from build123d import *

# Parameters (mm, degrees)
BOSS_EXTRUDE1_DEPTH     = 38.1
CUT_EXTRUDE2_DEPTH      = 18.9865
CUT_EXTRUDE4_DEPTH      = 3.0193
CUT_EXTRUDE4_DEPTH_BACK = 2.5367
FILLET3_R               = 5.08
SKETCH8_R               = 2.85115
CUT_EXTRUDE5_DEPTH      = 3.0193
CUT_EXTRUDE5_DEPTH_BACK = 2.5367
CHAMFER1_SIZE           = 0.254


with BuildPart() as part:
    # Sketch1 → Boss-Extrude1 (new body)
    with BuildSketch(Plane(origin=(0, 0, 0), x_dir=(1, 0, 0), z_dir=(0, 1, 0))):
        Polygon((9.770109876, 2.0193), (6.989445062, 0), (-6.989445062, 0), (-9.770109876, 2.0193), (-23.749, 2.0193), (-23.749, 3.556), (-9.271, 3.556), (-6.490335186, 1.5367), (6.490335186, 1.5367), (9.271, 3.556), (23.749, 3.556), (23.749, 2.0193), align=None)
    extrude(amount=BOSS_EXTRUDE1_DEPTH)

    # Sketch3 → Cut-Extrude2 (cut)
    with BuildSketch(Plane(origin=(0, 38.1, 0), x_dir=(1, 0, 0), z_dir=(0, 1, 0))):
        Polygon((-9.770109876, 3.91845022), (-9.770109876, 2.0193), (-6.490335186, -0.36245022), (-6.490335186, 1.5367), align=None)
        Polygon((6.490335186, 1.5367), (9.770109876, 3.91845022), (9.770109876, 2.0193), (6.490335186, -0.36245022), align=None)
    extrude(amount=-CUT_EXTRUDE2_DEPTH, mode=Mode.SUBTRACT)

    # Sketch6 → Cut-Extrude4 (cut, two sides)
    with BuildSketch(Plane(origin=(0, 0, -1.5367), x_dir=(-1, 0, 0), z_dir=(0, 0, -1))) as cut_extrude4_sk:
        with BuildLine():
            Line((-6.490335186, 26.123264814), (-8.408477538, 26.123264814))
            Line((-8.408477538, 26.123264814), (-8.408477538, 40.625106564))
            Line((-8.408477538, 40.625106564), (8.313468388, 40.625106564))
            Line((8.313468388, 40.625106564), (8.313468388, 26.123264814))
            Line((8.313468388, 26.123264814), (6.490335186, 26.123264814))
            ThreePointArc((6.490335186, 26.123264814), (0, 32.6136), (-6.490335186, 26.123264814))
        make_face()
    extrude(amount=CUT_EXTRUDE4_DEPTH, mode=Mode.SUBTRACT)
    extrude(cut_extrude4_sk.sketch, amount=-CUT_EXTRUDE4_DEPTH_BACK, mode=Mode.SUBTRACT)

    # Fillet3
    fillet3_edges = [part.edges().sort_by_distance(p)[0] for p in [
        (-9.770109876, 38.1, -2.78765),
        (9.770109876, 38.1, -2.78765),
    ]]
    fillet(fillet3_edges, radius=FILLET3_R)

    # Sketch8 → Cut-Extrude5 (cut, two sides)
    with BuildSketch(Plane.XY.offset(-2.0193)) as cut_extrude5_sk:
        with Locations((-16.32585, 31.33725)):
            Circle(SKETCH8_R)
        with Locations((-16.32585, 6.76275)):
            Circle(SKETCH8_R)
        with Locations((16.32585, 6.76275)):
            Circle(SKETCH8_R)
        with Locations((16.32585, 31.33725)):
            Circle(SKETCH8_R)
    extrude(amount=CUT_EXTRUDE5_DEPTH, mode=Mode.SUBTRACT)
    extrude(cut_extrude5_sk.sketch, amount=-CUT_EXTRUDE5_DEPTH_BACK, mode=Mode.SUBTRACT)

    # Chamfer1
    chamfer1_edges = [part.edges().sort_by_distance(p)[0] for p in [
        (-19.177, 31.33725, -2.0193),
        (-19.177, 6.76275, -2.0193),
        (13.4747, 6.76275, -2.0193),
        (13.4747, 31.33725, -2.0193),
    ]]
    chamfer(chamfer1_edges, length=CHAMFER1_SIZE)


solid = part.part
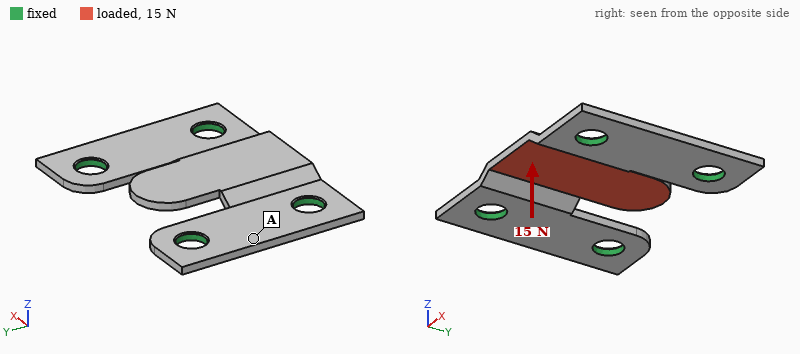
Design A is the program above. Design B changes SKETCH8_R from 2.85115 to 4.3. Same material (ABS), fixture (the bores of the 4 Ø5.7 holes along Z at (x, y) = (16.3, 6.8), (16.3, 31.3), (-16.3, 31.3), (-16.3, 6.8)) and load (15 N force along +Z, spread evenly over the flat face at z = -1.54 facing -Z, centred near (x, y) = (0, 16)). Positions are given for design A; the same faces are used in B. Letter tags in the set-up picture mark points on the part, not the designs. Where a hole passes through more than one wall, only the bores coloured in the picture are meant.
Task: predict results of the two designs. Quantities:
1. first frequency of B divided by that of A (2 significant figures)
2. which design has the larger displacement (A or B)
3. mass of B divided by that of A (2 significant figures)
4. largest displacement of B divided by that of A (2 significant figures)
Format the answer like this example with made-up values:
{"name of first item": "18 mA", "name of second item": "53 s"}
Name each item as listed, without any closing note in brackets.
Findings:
{"first frequency of B divided by that of A": "1.1", "which design has the larger displacement": "A", "mass of B divided by that of A": "0.91", "largest displacement of B divided by that of A": "0.91"}
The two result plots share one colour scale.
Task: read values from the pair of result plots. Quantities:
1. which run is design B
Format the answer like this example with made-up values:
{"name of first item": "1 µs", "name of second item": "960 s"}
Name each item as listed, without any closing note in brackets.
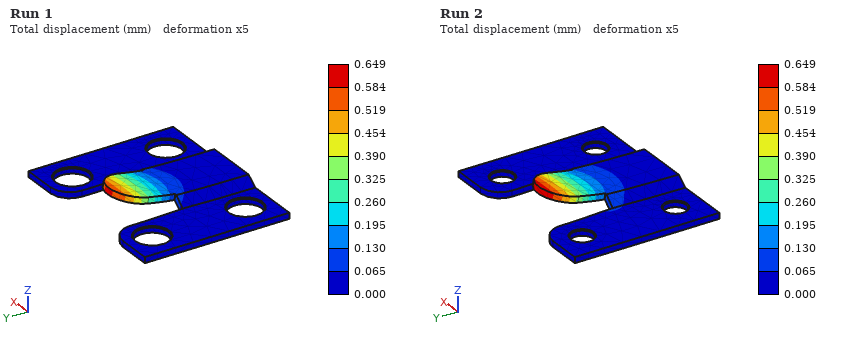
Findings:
{"which run is design B": "Run 1"}
